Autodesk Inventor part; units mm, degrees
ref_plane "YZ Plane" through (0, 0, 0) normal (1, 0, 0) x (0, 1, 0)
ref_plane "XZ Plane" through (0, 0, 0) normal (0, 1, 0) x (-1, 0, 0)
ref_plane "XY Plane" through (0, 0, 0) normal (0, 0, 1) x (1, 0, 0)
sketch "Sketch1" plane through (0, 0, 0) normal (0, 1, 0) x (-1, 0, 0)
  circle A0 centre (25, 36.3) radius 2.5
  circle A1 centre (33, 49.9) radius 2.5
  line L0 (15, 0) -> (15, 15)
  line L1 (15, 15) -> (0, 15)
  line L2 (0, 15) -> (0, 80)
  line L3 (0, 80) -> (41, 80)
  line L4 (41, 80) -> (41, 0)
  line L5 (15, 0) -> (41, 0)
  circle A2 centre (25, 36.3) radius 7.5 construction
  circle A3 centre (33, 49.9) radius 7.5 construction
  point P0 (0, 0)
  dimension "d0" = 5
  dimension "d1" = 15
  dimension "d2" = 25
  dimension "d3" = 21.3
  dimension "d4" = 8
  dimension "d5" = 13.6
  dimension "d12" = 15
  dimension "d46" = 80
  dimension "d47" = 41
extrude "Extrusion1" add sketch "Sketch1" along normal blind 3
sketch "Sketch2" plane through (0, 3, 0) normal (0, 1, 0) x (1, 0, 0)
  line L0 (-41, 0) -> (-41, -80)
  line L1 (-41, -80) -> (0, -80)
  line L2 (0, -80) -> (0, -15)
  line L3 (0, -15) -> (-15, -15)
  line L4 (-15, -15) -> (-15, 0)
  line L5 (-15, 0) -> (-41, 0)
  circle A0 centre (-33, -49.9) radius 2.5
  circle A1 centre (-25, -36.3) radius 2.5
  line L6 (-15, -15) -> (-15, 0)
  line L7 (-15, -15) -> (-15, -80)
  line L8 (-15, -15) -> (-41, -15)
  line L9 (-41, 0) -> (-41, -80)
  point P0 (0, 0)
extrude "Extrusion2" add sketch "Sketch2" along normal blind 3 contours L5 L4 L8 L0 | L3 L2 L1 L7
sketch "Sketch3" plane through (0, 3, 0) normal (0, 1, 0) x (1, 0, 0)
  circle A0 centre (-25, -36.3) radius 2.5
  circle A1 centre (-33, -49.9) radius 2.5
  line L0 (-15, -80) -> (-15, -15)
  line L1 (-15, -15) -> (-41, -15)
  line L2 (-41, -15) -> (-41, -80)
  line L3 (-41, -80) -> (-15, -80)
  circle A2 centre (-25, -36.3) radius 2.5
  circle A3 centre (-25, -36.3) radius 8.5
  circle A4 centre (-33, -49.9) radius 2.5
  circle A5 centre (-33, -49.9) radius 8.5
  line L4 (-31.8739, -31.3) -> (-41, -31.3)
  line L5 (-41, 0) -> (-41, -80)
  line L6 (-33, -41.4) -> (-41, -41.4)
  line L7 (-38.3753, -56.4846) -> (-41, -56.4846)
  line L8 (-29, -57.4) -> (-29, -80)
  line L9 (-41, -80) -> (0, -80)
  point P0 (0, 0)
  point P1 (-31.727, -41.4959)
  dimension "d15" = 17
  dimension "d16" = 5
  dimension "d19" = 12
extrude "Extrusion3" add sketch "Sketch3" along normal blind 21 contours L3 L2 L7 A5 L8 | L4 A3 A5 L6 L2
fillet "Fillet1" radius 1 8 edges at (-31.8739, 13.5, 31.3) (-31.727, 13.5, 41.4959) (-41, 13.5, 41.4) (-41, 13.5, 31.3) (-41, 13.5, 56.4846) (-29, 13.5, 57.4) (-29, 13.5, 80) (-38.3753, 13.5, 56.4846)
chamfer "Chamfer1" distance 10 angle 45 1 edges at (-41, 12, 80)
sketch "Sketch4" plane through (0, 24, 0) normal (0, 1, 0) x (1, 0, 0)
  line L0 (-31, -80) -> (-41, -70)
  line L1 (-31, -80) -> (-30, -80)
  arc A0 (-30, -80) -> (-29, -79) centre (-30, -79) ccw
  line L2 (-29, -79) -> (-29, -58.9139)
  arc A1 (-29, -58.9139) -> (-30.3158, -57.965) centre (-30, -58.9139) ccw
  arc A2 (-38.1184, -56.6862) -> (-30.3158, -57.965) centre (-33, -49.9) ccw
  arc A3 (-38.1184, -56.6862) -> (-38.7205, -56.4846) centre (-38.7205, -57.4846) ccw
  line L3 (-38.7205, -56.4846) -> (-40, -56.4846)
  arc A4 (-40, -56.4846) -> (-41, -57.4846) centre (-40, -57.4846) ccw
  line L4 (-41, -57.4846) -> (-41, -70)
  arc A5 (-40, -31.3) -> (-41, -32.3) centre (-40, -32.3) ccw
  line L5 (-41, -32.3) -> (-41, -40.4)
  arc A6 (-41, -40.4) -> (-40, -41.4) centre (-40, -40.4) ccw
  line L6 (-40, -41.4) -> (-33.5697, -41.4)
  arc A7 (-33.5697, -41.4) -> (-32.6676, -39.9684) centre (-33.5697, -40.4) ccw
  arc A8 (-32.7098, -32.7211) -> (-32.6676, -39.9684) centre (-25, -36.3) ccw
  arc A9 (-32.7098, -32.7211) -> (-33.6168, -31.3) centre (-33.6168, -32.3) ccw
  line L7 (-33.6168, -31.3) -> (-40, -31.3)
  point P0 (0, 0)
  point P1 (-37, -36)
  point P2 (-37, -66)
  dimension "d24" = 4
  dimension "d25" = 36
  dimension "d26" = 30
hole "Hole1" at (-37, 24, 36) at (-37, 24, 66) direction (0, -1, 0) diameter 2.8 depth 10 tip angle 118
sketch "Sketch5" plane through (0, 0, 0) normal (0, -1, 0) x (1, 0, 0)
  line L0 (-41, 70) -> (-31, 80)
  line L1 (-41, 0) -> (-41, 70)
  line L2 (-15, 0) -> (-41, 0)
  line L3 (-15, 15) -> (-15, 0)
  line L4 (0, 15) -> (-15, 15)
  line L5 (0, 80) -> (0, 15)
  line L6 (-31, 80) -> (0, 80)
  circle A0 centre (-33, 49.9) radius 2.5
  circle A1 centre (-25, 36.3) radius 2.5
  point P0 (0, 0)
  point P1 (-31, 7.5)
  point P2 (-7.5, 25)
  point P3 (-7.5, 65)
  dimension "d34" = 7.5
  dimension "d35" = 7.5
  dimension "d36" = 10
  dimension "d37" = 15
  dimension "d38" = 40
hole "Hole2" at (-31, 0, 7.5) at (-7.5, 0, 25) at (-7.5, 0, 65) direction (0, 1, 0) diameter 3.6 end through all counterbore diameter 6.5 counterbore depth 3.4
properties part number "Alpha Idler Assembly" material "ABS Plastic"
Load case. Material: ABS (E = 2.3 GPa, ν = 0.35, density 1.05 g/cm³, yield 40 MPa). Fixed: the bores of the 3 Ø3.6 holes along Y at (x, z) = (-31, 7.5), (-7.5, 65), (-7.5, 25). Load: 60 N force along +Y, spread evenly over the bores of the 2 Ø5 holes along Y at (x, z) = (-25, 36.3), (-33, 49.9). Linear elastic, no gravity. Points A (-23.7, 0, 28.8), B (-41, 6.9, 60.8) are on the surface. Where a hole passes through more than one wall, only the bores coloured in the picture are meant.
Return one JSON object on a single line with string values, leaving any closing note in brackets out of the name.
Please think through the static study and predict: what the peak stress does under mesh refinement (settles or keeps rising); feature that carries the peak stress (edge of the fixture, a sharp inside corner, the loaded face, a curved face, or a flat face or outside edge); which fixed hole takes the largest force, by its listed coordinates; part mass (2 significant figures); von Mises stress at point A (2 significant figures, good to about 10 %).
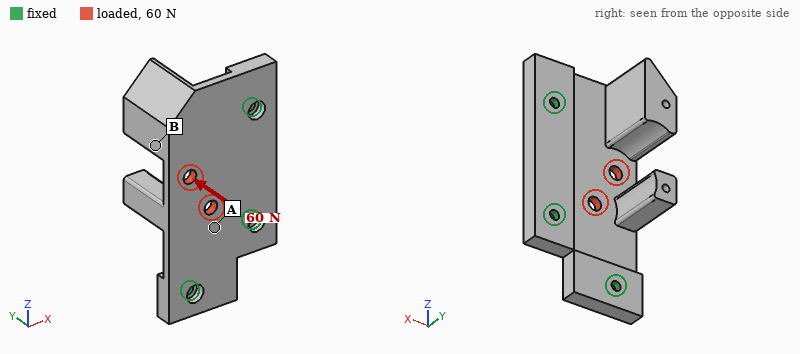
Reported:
{"what the peak stress does under mesh refinement": "keeps rising", "feature that carries the peak stress": "edge of the fixture", "which fixed hole takes the largest force, by its listed coordinates": "(-7.5, 65)", "part mass": "20 g", "von Mises stress at point A": "4.6 MPa"}
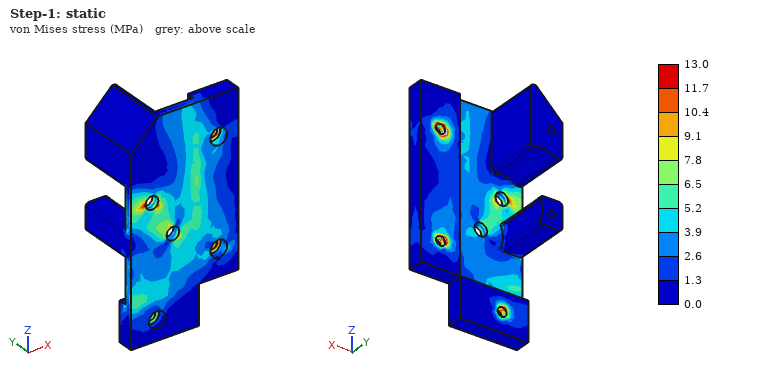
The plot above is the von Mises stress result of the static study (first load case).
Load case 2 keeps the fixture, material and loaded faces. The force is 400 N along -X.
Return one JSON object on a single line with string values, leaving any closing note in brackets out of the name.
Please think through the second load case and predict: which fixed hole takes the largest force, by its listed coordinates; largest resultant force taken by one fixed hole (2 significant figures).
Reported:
{"which fixed hole takes the largest force, by its listed coordinates": "(-7.5, 25)", "largest resultant force taken by one fixed hole": "190 N"}
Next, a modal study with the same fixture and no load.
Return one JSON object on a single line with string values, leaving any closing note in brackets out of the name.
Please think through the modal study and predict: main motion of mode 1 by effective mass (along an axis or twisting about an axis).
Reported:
{"main motion of mode 1 by effective mass": "along Y"}
